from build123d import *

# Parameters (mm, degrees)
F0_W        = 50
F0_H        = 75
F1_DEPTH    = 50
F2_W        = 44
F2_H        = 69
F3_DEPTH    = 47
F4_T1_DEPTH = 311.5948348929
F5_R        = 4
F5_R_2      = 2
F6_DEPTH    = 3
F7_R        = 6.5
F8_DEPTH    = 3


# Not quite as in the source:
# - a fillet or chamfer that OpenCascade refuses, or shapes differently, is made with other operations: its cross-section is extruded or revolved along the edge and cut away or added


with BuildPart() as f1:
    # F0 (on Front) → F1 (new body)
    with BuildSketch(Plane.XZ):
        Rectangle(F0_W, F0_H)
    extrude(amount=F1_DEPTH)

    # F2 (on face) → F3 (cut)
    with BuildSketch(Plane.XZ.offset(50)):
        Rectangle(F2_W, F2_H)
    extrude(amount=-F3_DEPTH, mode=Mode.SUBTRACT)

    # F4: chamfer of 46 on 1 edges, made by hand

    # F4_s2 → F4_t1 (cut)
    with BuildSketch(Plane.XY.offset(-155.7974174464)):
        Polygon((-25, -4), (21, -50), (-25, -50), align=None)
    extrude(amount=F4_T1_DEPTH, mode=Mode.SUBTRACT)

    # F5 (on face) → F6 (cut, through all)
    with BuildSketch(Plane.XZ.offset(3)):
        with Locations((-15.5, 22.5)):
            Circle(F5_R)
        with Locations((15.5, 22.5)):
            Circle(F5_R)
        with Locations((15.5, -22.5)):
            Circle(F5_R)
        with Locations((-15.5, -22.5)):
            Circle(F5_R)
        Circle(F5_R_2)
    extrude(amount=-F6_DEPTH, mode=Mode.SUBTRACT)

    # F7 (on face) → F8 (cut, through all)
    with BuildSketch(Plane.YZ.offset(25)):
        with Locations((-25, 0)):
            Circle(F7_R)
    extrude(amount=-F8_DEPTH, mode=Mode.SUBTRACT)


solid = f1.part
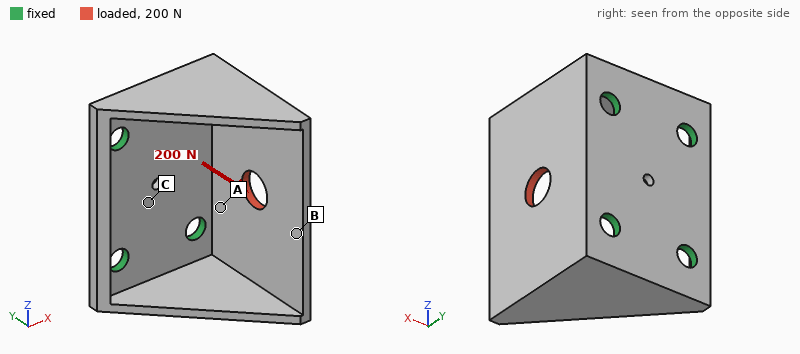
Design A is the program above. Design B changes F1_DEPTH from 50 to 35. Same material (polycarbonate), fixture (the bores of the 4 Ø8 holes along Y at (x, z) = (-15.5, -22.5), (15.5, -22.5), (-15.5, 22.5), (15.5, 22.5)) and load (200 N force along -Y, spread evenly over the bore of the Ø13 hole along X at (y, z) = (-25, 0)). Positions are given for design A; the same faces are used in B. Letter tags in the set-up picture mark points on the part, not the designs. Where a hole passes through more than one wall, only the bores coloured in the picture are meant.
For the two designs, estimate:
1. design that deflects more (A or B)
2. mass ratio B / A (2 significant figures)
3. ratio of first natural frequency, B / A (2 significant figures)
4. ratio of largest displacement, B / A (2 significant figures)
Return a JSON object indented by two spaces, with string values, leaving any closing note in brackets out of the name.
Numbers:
{
  "design that deflects more": "B",
  "mass ratio B / A": "0.85",
  "ratio of first natural frequency, B / A": "1.5",
  "ratio of largest displacement, B / A": "1.2"
}
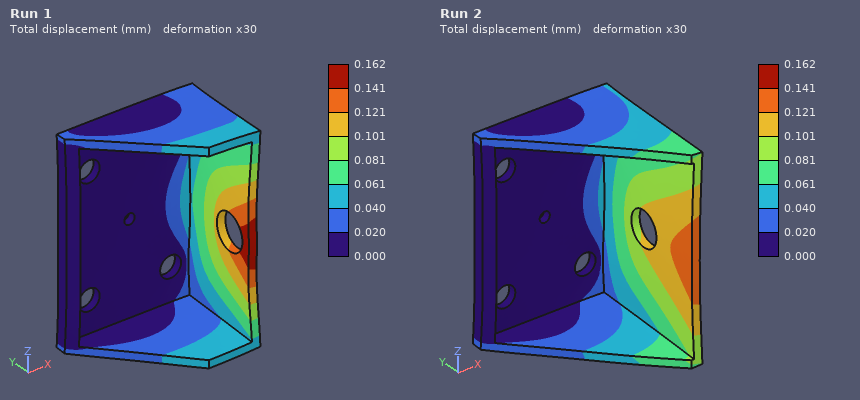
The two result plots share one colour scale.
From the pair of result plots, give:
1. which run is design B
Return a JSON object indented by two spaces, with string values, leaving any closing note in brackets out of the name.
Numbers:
{
  "which run is design B": "Run 1"
}
